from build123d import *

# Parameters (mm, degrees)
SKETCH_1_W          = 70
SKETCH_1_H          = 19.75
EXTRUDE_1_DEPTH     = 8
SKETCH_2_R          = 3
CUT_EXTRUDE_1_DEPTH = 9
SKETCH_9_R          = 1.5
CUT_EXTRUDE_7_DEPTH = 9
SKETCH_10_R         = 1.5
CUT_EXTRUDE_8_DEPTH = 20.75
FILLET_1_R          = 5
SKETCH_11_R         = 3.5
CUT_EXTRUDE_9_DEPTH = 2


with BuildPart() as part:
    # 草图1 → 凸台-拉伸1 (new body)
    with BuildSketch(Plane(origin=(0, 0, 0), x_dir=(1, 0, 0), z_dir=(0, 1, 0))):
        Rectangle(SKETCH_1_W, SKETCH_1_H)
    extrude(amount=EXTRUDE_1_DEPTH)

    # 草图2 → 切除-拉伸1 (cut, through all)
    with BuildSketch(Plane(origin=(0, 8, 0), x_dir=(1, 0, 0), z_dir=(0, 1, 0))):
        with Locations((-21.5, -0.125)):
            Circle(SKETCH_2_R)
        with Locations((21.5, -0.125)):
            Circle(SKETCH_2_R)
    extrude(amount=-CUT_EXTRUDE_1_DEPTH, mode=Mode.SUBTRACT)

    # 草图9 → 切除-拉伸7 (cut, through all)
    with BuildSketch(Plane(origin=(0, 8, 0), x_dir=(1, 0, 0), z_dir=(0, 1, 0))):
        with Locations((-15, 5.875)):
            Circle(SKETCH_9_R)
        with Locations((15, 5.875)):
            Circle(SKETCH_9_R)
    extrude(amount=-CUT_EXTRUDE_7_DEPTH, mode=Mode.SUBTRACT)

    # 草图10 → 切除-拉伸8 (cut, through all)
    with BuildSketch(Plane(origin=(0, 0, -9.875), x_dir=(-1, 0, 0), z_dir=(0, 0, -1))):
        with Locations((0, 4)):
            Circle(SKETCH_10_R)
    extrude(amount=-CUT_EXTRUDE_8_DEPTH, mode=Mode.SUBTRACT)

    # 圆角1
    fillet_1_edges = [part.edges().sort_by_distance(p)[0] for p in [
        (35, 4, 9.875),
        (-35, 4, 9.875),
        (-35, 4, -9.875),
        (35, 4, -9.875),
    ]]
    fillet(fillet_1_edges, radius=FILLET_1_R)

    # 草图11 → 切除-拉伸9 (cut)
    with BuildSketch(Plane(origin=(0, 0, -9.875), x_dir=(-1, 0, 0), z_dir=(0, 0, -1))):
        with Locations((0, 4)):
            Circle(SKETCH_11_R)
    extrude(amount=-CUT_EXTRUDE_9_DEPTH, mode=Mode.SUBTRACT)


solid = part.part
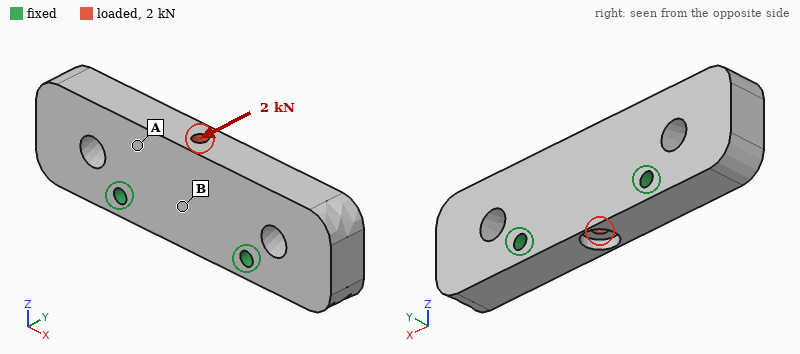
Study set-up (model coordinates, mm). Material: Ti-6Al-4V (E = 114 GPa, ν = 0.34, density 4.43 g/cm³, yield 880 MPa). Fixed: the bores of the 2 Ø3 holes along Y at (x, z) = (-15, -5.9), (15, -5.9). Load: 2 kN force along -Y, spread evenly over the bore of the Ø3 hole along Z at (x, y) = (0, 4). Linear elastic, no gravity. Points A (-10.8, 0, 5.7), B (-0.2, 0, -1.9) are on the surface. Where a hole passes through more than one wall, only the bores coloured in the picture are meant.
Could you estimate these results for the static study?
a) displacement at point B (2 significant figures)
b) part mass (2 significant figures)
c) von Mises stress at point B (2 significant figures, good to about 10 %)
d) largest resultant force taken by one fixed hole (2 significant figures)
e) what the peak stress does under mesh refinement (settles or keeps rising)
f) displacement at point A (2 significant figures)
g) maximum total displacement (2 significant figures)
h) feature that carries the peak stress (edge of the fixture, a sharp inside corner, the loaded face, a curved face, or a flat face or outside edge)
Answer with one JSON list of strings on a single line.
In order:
["9.1 µm", "45 g", "42 MPa", "1.0 kN", "keeps rising", "9.9 µm", "18 µm", "edge of the fixture"]
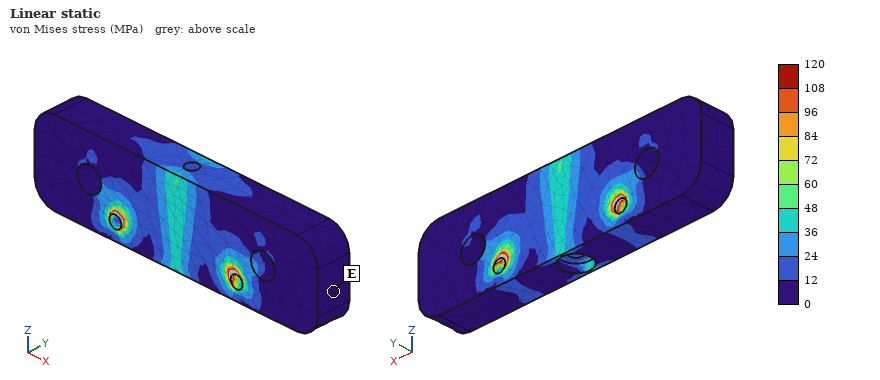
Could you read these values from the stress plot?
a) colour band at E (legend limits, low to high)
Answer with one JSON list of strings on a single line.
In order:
["0 to 12 MPa"]
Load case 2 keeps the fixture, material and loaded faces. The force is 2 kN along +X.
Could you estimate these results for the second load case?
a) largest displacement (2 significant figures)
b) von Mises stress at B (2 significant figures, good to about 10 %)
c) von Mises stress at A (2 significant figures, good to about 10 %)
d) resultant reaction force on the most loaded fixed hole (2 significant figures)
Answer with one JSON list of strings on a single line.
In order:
["2.9 µm", "8.3 MPa", "3.3 MPa", "1.1 kN"]
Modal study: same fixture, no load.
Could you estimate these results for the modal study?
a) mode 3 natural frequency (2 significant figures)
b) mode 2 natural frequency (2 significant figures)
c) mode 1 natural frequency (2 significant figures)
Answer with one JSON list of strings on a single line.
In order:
["15 kHz", "11 kHz", "11 kHz"]
